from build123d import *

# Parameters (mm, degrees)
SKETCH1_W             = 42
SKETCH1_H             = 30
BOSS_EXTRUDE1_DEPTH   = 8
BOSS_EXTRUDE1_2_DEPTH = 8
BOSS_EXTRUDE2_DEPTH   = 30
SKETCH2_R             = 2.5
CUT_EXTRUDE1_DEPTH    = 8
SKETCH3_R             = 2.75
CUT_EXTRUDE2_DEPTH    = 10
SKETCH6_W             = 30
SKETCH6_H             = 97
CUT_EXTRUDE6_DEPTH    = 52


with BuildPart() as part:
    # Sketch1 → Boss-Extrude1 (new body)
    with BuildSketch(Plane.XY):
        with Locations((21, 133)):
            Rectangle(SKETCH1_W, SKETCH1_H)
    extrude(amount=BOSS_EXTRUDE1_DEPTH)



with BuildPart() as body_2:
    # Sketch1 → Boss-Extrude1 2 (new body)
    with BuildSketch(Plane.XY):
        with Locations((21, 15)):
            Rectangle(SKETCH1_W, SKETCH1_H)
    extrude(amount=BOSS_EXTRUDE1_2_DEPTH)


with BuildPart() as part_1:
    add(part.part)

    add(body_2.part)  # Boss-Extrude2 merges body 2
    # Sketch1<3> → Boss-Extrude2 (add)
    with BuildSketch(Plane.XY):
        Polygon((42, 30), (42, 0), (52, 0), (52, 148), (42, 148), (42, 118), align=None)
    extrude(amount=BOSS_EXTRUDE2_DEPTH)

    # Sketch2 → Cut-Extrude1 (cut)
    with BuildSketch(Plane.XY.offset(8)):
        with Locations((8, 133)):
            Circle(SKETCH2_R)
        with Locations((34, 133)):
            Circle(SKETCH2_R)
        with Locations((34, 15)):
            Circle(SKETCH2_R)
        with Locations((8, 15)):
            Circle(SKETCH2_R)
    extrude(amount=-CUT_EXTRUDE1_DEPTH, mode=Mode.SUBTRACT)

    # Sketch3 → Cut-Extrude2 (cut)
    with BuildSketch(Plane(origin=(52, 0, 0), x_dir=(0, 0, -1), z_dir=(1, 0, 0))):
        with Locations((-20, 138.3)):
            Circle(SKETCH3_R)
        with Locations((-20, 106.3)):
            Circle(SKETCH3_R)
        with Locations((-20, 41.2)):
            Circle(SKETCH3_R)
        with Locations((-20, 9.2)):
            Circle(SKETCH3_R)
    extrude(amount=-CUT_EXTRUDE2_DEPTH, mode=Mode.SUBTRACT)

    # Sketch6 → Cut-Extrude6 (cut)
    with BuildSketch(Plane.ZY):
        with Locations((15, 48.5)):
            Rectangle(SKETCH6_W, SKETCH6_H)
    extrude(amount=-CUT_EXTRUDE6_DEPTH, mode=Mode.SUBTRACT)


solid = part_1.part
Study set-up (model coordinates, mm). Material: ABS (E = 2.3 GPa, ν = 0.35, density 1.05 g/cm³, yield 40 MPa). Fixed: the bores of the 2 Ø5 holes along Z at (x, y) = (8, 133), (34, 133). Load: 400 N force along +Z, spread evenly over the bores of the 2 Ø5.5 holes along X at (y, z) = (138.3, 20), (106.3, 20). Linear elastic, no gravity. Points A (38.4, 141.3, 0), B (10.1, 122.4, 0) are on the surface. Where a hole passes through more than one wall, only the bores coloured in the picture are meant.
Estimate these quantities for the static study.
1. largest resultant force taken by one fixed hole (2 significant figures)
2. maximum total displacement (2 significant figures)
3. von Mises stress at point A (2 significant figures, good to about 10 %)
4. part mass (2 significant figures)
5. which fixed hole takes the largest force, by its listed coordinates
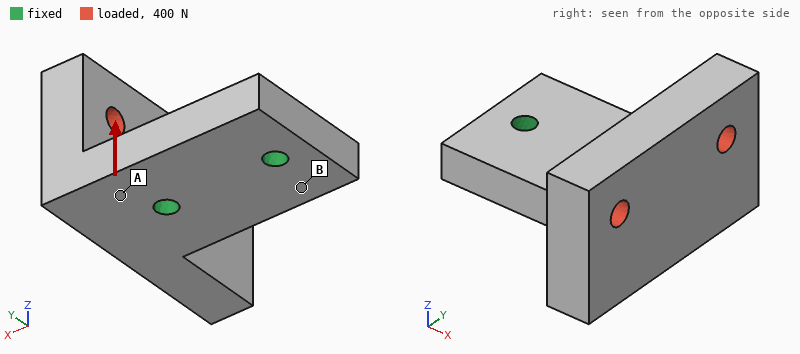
460 N
0.89 mm
8.5 MPa
26 g
(34, 133)
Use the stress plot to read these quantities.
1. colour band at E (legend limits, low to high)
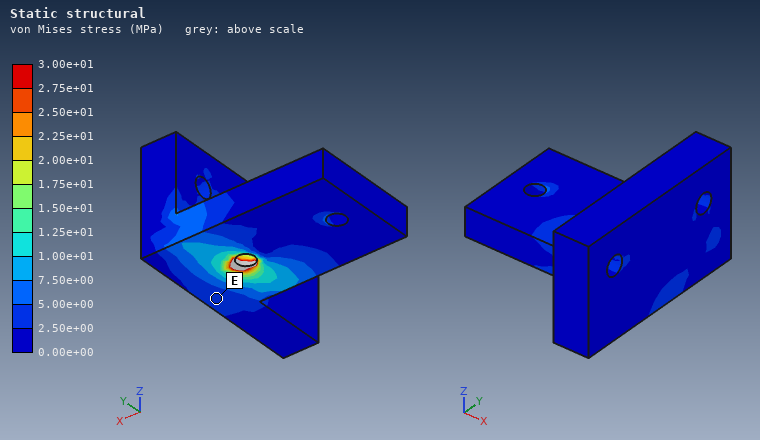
2.50e+00 to 5.00e+00 MPa
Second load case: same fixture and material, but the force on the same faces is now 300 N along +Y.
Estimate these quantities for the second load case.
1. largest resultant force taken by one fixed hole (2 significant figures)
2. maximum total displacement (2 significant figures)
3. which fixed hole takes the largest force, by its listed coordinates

410 N
0.64 mm
(34, 133)
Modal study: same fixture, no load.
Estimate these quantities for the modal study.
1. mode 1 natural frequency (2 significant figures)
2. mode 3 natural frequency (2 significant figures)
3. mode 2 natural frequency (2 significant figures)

940 Hz
2000 Hz
1200 Hz
